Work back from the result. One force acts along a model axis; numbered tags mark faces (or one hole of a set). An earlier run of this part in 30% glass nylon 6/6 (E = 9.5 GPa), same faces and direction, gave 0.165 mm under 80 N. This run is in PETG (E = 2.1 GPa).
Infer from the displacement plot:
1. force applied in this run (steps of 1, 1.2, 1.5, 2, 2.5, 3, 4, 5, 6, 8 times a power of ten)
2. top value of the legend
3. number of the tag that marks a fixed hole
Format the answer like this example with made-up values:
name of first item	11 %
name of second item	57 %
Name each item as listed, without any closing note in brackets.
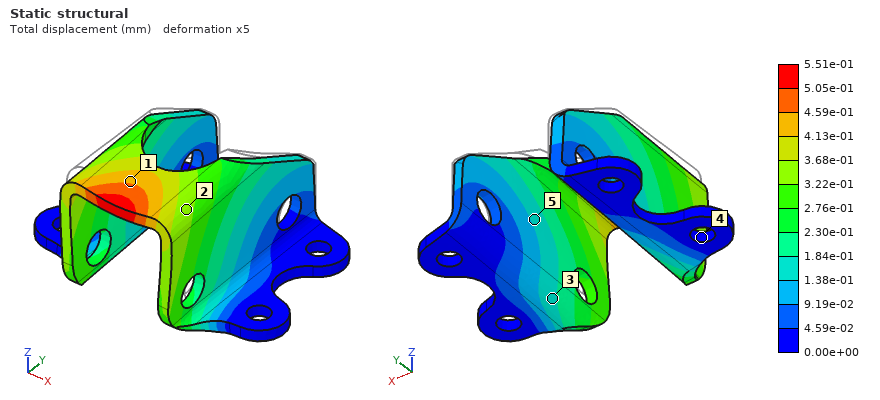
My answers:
force applied in this run	60 N
top value of the legend	5.51e-01 mm
number of the tag that marks a fixed hole	4
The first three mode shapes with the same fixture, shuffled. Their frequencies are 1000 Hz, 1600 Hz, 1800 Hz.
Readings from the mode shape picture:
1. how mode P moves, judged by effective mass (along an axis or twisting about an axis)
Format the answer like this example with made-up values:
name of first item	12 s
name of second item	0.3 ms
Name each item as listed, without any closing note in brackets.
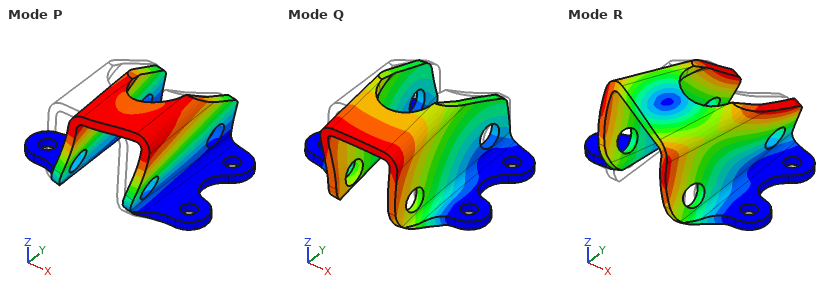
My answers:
how mode P moves, judged by effective mass	along X
